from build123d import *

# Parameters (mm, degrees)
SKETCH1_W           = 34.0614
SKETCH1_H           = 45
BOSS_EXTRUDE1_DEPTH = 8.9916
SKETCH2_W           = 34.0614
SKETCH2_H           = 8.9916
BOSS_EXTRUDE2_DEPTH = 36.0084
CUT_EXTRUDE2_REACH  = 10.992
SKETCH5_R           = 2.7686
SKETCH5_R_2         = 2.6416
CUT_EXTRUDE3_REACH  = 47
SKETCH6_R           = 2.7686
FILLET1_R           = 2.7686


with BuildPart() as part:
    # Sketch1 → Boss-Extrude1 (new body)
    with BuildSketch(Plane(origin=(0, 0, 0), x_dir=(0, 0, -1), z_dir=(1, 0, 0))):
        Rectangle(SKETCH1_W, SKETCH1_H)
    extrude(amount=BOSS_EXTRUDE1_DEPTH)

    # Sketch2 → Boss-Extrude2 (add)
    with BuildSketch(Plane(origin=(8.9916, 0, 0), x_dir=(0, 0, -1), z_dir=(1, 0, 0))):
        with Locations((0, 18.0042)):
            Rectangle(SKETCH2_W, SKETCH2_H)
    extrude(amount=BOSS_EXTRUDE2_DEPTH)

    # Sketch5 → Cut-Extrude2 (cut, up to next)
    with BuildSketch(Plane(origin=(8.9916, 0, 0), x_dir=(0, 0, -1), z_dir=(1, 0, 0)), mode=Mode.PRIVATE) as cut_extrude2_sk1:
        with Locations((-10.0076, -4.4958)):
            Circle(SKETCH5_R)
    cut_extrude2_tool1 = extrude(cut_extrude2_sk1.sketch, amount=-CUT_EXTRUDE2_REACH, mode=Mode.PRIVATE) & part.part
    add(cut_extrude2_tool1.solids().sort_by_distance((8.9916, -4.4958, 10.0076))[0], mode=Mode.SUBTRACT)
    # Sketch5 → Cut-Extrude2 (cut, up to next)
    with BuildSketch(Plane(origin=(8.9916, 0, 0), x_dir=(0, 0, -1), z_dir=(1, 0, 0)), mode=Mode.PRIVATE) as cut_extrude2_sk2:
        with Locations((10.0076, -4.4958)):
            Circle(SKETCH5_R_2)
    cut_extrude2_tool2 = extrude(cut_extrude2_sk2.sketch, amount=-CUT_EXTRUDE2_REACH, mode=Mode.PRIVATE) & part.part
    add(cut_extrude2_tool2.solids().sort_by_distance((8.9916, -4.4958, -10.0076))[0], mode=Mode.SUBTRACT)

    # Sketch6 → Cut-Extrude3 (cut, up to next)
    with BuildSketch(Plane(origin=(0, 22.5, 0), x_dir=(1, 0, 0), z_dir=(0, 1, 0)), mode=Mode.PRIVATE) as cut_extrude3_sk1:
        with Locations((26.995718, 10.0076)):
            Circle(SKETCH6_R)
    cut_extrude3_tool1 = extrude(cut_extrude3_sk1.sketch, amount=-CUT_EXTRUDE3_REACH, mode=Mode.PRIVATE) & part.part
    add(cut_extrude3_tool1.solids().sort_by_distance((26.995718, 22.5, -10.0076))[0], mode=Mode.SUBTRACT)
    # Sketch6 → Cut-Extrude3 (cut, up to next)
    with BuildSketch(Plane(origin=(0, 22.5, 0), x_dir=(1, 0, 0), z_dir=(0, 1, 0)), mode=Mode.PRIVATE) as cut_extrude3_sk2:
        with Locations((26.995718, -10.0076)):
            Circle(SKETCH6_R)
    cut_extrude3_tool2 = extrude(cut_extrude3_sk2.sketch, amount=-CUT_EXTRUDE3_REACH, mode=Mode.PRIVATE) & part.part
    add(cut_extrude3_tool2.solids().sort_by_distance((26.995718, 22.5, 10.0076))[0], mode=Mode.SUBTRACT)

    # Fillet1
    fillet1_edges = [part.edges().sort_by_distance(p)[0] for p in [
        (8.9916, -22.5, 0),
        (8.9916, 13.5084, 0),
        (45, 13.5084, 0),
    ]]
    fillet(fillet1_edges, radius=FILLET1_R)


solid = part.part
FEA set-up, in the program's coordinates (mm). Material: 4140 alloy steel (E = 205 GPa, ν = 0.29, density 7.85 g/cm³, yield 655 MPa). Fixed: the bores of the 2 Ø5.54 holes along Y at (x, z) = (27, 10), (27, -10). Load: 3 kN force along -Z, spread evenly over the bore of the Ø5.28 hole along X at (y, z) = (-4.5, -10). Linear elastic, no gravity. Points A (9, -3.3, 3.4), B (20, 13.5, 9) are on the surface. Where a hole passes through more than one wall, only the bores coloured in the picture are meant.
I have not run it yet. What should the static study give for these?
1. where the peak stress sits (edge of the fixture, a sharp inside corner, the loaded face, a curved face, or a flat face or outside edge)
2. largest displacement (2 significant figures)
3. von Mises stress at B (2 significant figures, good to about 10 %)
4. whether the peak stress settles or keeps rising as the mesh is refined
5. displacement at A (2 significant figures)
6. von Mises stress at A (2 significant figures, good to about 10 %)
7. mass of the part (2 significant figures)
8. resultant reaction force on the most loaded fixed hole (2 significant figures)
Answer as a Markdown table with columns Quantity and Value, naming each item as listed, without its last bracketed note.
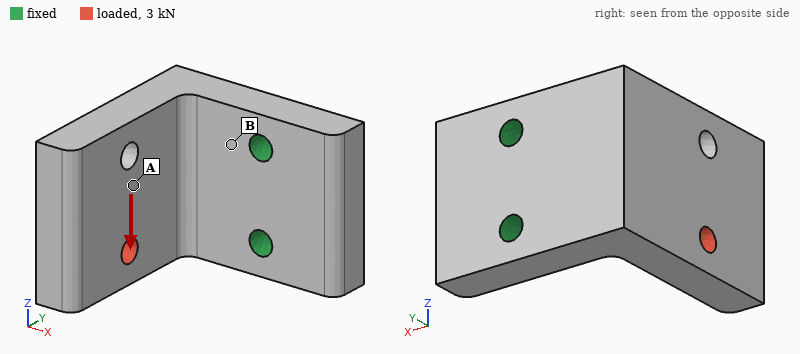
| Quantity | Value |
|---|---|
| where the peak stress sits | edge of the fixture |
| largest displacement | 66 µm |
| von Mises stress at B | 88 MPa |
| whether the peak stress settles or keeps rising as the mesh is refined | keeps rising |
| displacement at A | 35 µm |
| von Mises stress at A | 26 MPa |
| mass of the part | 190 g |
| resultant reaction force on the most loaded fixed hole | 4.1 kN |
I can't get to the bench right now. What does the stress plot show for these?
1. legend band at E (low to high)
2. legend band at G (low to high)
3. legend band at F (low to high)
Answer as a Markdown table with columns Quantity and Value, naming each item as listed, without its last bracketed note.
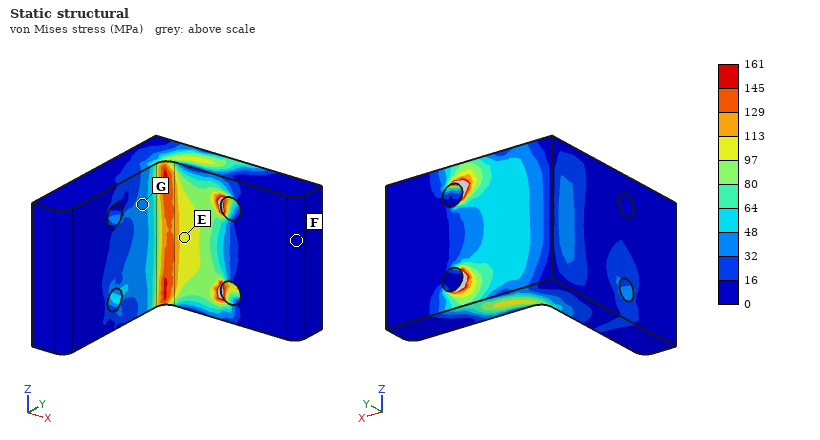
| Quantity | Value |
|---|---|
| legend band at E | 97 to 113 MPa |
| legend band at G | 32 to 48 MPa |
| legend band at F | 0 to 16 MPa |
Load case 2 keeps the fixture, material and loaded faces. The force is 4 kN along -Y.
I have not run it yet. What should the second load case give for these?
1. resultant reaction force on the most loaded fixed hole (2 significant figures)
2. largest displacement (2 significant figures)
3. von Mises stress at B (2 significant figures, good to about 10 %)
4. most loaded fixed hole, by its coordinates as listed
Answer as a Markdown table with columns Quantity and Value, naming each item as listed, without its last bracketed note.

| Quantity | Value |
|---|---|
| resultant reaction force on the most loaded fixed hole | 3.5 kN |
| largest displacement | 0.12 mm |
| von Mises stress at B | 130 MPa |
| most loaded fixed hole, by its coordinates as listed | (27, -10) |
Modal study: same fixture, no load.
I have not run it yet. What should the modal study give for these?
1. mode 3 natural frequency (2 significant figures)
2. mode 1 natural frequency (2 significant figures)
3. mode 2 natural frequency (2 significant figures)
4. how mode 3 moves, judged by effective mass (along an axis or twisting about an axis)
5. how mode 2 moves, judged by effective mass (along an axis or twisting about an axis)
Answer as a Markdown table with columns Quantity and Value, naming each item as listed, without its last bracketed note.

| Quantity | Value |
|---|---|
| mode 3 natural frequency | 7800 Hz |
| mode 1 natural frequency | 2600 Hz |
| mode 2 natural frequency | 4300 Hz |
| how mode 3 moves, judged by effective mass | along Y |
| how mode 2 moves, judged by effective mass | along Z |
